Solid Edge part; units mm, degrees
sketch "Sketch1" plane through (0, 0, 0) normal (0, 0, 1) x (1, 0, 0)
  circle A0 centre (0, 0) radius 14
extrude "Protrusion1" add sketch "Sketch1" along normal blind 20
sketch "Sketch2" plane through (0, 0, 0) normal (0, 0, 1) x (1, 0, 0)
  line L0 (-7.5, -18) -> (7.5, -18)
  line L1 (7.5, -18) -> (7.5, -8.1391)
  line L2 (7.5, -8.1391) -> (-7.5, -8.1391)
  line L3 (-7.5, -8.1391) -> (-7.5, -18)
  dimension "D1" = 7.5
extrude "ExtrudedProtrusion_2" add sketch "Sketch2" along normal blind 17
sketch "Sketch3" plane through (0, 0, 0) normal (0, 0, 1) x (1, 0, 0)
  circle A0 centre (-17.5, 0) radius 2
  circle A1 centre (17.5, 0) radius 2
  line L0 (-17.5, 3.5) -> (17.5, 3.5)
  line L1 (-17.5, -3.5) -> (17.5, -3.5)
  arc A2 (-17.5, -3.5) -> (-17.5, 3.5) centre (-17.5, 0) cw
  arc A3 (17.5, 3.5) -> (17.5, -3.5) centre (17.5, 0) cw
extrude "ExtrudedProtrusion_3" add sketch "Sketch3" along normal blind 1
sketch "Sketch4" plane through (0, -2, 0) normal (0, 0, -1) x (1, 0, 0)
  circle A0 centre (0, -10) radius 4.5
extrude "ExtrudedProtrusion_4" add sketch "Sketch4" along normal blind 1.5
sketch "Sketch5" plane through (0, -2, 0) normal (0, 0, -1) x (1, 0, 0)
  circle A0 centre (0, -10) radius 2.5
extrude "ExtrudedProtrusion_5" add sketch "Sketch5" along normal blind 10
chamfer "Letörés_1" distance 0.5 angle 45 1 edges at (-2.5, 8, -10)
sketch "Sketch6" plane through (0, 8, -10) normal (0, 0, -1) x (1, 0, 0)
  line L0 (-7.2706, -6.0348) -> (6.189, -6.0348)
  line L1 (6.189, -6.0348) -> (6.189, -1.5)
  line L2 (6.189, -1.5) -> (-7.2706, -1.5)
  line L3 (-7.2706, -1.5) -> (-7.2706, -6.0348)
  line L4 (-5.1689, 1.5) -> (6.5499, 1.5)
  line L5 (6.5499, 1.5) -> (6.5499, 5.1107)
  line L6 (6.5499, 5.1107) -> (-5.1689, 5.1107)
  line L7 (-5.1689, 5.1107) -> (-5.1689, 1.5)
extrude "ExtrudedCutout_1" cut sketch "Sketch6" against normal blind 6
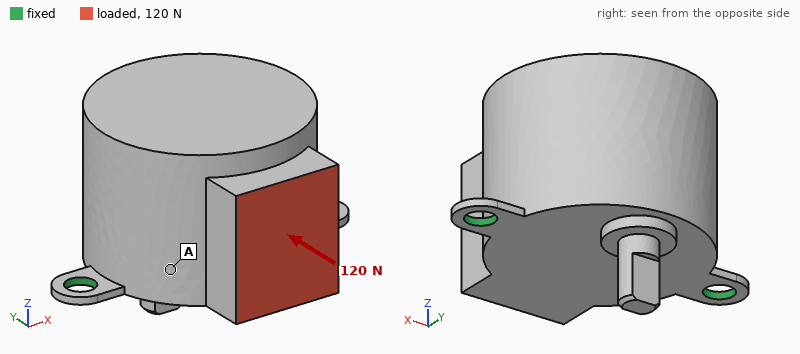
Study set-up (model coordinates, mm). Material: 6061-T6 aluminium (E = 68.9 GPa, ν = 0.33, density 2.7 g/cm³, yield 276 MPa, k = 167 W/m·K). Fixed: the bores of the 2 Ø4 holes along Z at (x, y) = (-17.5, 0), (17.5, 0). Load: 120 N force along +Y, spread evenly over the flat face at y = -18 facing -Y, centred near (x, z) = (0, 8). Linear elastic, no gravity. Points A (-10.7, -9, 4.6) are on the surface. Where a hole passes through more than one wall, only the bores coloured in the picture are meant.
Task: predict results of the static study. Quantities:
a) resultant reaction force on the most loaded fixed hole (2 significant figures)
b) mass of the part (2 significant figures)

60 N
37 g
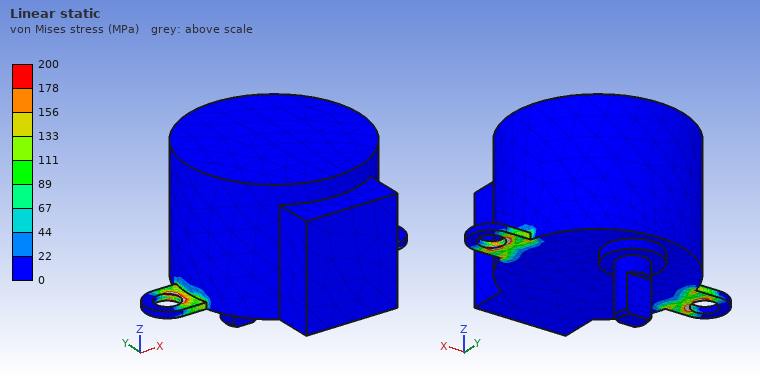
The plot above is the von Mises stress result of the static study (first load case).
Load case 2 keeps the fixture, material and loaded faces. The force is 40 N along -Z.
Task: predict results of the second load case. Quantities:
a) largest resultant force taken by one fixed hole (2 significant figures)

24 N
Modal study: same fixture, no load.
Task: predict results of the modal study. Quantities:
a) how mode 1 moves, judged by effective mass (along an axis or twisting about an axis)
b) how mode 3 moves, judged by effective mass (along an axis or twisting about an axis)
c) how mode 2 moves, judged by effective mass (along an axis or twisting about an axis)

along Y
along X
along Z
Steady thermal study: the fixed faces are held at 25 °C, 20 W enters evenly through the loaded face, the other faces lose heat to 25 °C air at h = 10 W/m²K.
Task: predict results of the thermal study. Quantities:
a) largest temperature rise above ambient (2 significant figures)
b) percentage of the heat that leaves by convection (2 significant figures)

36 K
5.0 %
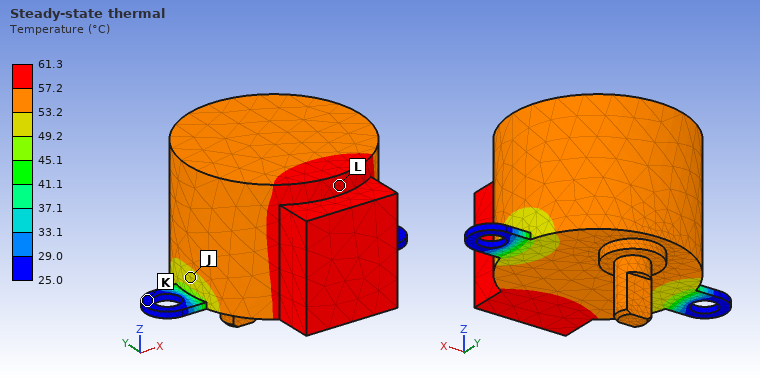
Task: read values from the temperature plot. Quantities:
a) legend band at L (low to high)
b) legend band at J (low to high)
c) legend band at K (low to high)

57.2 to 61.3 °C
49.2 to 53.2 °C
25.0 to 29.0 °C
